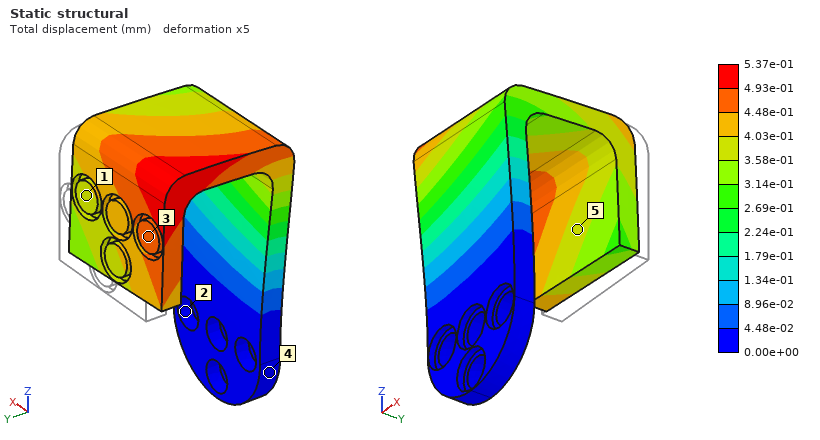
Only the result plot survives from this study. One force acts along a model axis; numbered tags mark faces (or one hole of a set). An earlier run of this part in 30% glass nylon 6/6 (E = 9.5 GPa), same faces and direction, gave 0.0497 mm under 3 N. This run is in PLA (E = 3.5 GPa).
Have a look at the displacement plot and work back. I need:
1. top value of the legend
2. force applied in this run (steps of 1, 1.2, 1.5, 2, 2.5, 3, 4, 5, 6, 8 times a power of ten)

5.37e-01 mm
12 N
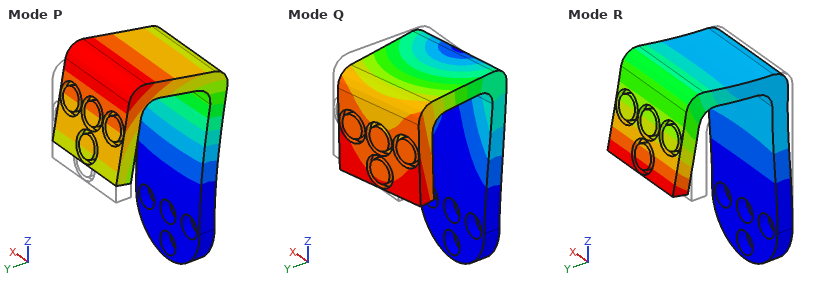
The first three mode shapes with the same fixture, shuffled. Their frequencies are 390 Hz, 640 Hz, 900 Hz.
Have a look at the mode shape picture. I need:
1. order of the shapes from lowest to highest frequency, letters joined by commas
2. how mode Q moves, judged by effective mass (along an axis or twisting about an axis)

P, Q, R
along X
